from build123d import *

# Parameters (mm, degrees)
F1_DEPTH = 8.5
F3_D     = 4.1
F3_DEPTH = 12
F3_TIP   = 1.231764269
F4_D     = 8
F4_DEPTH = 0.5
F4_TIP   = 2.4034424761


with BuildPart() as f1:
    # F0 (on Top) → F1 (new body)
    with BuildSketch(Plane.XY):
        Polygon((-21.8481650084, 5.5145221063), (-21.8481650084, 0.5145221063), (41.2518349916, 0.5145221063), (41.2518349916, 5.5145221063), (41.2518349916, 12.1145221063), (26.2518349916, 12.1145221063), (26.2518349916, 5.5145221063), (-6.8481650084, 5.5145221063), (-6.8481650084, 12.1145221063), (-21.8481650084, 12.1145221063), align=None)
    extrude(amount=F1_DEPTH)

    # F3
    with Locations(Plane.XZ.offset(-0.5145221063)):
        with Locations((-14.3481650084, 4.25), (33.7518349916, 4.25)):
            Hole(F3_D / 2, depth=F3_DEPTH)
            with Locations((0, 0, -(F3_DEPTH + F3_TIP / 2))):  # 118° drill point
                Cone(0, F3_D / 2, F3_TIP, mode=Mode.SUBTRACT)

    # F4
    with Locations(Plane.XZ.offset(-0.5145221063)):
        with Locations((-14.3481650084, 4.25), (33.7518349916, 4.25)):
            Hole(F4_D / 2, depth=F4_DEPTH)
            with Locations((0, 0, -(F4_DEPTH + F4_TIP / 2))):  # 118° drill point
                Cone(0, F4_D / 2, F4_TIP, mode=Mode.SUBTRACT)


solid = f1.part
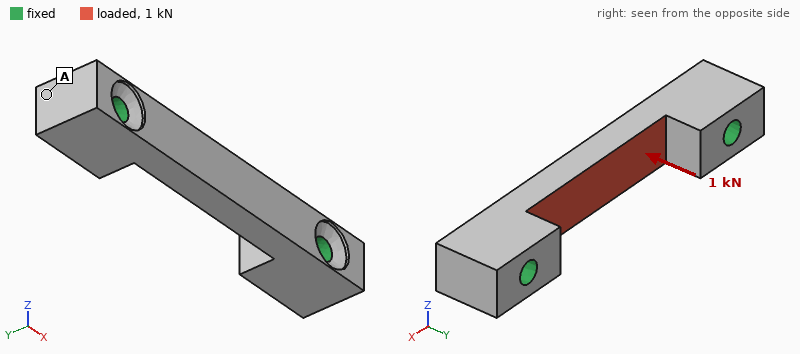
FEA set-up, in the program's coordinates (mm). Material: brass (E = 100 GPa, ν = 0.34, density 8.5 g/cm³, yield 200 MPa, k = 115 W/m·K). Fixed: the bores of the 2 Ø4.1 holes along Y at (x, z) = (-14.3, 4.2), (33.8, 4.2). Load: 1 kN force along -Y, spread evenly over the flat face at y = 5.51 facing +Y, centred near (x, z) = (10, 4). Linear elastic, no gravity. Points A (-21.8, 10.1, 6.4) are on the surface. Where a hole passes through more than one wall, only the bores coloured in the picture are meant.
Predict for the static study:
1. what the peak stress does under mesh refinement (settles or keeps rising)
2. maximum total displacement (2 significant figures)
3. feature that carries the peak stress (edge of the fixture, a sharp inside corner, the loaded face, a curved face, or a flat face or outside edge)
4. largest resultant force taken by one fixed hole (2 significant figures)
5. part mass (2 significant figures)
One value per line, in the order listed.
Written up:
keeps rising
24 µm
edge of the fixture
550 N
34 g
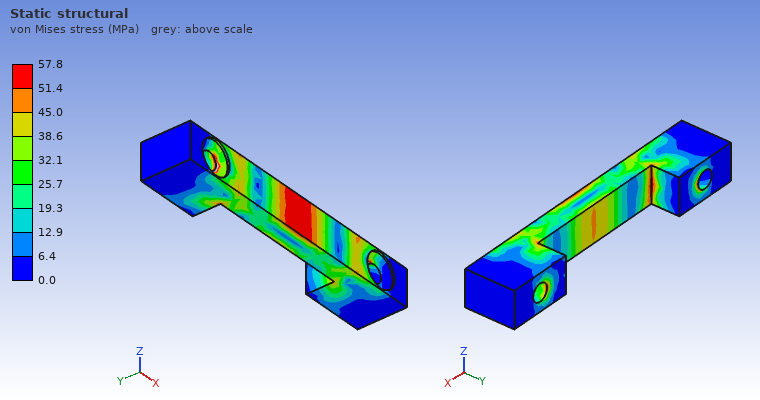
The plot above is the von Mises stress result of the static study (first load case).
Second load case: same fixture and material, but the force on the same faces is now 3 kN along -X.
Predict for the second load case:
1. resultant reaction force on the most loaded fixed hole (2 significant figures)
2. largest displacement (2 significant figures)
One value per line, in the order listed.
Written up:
1.5 kN
7.0 µm
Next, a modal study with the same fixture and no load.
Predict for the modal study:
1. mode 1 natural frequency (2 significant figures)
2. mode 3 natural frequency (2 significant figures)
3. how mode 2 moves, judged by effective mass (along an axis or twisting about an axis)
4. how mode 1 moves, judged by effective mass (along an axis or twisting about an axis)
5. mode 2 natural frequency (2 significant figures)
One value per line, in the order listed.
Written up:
11 kHz
23 kHz
along Z
along Y
12 kHz
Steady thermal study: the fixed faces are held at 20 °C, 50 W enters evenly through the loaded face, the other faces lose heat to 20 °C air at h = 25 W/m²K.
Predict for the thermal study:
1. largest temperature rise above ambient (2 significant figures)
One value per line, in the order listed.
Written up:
67 K
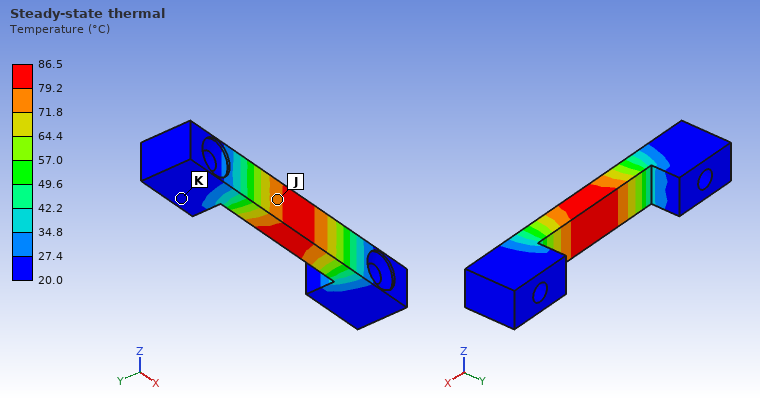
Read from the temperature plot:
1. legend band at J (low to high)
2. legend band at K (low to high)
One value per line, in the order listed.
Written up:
71.8 to 79.2 °C
20.0 to 27.4 °C
